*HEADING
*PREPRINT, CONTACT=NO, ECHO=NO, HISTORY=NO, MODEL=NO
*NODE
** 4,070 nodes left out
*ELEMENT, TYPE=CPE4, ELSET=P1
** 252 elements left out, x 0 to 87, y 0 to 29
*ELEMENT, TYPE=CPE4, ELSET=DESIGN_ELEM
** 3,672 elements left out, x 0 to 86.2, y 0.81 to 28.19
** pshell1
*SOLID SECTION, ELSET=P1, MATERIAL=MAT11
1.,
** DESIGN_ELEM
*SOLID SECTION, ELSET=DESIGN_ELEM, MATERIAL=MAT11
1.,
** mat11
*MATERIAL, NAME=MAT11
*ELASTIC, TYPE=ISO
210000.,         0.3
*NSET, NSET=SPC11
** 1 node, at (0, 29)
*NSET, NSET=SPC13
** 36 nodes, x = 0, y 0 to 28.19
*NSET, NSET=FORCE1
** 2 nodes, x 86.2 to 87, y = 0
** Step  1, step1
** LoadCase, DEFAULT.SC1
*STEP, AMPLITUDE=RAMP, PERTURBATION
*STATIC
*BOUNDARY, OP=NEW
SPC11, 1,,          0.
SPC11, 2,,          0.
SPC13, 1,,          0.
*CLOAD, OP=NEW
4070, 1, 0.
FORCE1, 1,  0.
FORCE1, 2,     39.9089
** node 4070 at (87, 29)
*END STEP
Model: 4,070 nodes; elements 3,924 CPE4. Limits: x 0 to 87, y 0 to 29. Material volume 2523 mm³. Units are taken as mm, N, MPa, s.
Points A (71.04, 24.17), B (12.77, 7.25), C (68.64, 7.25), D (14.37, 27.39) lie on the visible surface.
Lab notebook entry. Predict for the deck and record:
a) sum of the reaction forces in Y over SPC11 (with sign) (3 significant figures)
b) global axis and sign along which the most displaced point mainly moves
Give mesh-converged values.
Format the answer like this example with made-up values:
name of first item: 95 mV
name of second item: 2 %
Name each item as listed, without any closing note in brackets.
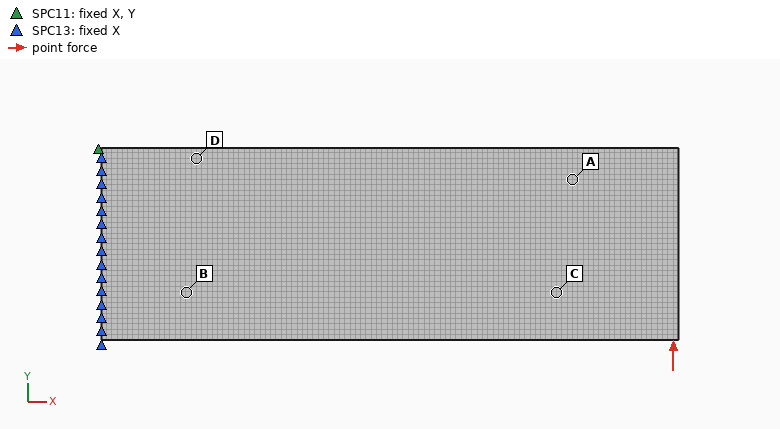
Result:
sum of the reaction forces in Y over SPC11 (with sign): -79.8 N
global axis and sign along which the most displaced point mainly moves: +Y
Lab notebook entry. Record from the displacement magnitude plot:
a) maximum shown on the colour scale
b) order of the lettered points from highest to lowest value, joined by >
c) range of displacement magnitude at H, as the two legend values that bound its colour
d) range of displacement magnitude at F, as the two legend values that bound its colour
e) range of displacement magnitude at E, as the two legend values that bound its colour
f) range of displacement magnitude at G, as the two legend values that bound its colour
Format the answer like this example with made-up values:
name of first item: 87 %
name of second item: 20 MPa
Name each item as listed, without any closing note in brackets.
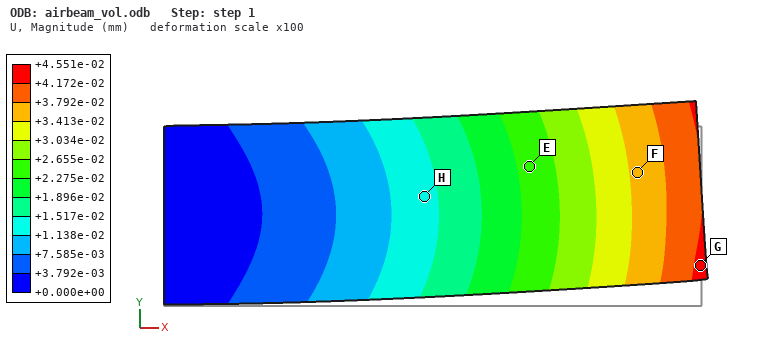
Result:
maximum shown on the colour scale: +4.551e-02 mm
order of the lettered points from highest to lowest value, joined by >: G > F > E > H
range of displacement magnitude at H, as the two legend values that bound its colour: +1.138e-02 to +1.517e-02 mm
range of displacement magnitude at F, as the two legend values that bound its colour: +3.413e-02 to +3.792e-02 mm
range of displacement magnitude at E, as the two legend values that bound its colour: +2.275e-02 to +2.655e-02 mm
range of displacement magnitude at G, as the two legend values that bound its colour: +4.172e-02 to +4.551e-02 mm
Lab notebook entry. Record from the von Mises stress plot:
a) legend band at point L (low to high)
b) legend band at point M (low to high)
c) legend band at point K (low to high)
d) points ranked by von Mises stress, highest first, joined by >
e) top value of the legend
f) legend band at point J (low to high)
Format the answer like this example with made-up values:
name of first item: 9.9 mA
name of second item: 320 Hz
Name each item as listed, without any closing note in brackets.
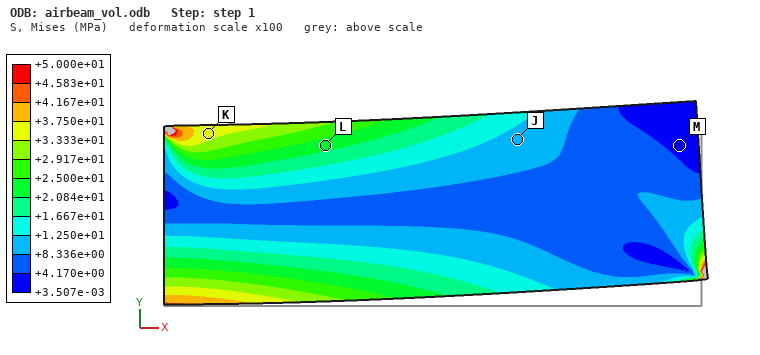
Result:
legend band at point L: +2.084e+01 to +2.500e+01 MPa
legend band at point M: +3.507e-03 to +4.170e+00 MPa
legend band at point K: +3.333e+01 to +3.750e+01 MPa
points ranked by von Mises stress, highest first, joined by >: K > L > J > M
top value of the legend: +5.000e+01 MPa
legend band at point J: +8.336e+00 to +1.250e+01 MPa
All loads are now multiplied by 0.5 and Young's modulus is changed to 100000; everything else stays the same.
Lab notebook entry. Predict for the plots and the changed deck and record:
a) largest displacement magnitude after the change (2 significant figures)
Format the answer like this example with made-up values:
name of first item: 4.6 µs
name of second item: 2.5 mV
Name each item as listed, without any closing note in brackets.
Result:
largest displacement magnitude after the change: 0.048 mm
